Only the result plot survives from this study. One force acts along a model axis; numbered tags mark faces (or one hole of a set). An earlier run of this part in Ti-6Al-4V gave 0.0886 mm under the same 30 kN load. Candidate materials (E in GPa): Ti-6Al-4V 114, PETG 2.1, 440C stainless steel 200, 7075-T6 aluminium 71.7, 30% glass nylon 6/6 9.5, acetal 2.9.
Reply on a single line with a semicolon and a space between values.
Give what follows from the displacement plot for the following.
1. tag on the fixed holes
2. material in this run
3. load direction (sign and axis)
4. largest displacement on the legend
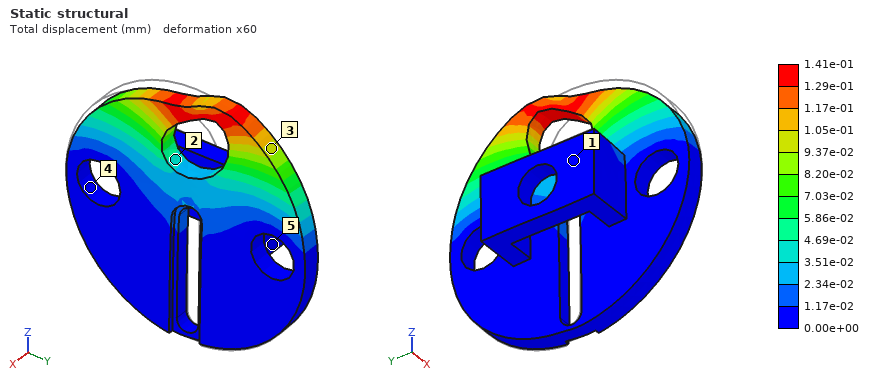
4; 7075-T6 aluminium; +Y; 1.41e-01 mm
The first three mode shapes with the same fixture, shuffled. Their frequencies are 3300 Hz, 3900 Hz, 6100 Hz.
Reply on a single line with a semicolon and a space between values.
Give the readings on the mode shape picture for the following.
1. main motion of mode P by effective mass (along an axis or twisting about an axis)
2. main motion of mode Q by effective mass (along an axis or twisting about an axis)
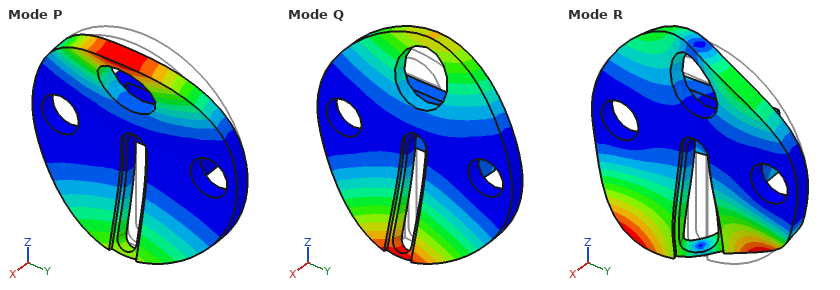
along X; twisting about Y
